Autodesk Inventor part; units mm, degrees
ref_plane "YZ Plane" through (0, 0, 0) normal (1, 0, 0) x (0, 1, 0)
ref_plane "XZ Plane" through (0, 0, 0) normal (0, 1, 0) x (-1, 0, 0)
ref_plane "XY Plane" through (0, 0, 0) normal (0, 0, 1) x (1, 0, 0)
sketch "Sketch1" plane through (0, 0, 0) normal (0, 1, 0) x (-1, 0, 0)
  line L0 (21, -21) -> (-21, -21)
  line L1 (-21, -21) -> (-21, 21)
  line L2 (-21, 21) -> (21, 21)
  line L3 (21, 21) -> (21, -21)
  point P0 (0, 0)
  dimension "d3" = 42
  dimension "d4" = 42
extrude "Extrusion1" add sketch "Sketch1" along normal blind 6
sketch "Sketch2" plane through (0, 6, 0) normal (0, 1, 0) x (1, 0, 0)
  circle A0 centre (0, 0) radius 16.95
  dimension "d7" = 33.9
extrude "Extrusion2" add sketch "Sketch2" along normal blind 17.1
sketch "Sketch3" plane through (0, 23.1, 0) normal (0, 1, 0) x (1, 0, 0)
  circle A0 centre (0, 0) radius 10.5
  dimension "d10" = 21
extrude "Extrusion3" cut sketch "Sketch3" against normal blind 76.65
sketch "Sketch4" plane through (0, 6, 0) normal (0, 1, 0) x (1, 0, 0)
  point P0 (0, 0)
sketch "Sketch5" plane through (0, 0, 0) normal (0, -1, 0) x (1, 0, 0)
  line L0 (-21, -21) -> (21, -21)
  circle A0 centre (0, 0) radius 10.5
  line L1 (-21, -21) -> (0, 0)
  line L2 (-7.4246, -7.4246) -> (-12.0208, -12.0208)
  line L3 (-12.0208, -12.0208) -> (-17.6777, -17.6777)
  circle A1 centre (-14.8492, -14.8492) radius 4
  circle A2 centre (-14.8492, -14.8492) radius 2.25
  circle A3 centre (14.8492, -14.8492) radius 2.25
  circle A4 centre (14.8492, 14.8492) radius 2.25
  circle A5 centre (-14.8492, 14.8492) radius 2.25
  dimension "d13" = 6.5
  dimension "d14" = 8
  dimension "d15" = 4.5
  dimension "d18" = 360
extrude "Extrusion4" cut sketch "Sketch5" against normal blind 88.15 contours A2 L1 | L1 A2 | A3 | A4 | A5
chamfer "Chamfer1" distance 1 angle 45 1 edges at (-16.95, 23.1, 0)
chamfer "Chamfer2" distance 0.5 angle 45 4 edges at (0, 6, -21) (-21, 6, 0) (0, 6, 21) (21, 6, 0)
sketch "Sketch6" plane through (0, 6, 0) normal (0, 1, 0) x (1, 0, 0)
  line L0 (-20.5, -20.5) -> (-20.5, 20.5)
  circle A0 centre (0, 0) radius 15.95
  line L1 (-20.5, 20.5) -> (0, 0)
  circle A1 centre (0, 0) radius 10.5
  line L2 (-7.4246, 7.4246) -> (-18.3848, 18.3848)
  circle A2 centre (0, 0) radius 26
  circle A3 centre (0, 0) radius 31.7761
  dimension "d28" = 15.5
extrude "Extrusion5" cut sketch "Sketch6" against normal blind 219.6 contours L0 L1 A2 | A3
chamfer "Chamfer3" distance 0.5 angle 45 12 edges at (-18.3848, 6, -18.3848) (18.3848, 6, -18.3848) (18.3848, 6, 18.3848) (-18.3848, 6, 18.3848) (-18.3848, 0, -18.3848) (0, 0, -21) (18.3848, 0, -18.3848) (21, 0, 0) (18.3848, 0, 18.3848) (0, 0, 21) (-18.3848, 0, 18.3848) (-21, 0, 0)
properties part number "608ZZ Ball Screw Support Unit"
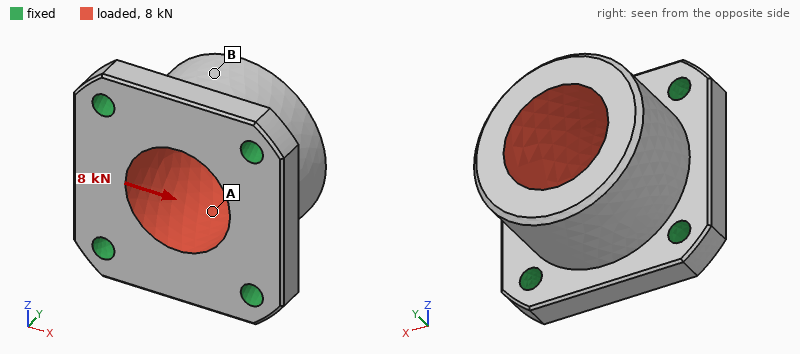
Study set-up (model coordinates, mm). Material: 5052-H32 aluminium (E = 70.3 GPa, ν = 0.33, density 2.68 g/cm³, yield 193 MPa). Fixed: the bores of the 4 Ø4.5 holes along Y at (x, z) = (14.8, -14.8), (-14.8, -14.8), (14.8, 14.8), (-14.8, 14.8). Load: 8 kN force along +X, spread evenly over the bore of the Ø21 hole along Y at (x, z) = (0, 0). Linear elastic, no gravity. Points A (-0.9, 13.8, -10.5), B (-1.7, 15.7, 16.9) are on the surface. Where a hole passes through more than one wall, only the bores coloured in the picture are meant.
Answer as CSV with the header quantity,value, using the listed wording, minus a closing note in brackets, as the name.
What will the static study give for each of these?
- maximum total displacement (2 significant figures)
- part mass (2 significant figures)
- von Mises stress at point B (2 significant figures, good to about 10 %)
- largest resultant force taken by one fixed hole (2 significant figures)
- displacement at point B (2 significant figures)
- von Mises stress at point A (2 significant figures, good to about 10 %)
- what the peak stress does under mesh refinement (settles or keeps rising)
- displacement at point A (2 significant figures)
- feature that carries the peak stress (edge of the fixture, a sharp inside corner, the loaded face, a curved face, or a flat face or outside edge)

quantity,value
maximum total displacement,20 µm
part mass,46 g
von Mises stress at point B,9.7 MPa
largest resultant force taken by one fixed hole,2.4 kN
displacement at point B,12 µm
von Mises stress at point A,31 MPa
what the peak stress does under mesh refinement,keeps rising
displacement at point A,11 µm
feature that carries the peak stress,edge of the fixture
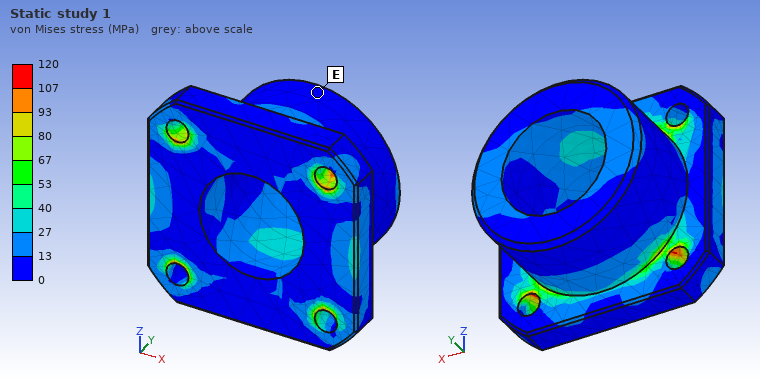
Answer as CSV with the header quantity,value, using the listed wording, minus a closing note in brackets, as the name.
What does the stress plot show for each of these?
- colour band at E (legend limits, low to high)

quantity,value
colour band at E,0 to 13 MPa
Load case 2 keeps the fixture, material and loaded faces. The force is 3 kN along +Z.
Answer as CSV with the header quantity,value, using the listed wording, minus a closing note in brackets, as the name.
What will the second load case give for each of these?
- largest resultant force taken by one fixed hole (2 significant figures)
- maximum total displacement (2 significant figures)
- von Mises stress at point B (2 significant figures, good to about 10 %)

quantity,value
largest resultant force taken by one fixed hole,890 N
maximum total displacement,7.5 µm
von Mises stress at point B,3.5 MPa
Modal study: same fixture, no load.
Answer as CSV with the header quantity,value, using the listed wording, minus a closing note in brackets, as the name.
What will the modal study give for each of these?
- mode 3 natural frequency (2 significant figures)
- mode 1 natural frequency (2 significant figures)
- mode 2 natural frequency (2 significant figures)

quantity,value
mode 3 natural frequency,24 kHz
mode 1 natural frequency,20 kHz
mode 2 natural frequency,20 kHz
